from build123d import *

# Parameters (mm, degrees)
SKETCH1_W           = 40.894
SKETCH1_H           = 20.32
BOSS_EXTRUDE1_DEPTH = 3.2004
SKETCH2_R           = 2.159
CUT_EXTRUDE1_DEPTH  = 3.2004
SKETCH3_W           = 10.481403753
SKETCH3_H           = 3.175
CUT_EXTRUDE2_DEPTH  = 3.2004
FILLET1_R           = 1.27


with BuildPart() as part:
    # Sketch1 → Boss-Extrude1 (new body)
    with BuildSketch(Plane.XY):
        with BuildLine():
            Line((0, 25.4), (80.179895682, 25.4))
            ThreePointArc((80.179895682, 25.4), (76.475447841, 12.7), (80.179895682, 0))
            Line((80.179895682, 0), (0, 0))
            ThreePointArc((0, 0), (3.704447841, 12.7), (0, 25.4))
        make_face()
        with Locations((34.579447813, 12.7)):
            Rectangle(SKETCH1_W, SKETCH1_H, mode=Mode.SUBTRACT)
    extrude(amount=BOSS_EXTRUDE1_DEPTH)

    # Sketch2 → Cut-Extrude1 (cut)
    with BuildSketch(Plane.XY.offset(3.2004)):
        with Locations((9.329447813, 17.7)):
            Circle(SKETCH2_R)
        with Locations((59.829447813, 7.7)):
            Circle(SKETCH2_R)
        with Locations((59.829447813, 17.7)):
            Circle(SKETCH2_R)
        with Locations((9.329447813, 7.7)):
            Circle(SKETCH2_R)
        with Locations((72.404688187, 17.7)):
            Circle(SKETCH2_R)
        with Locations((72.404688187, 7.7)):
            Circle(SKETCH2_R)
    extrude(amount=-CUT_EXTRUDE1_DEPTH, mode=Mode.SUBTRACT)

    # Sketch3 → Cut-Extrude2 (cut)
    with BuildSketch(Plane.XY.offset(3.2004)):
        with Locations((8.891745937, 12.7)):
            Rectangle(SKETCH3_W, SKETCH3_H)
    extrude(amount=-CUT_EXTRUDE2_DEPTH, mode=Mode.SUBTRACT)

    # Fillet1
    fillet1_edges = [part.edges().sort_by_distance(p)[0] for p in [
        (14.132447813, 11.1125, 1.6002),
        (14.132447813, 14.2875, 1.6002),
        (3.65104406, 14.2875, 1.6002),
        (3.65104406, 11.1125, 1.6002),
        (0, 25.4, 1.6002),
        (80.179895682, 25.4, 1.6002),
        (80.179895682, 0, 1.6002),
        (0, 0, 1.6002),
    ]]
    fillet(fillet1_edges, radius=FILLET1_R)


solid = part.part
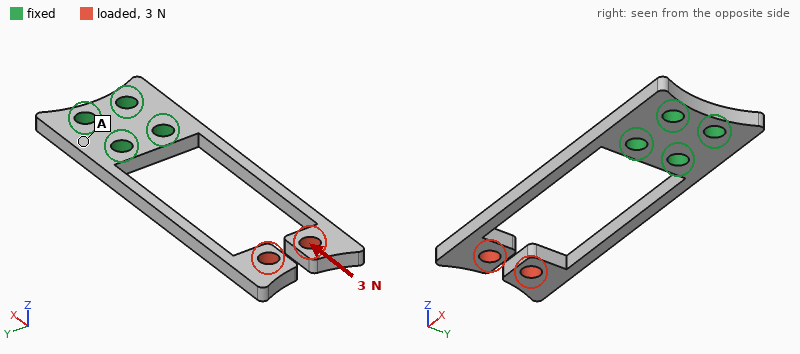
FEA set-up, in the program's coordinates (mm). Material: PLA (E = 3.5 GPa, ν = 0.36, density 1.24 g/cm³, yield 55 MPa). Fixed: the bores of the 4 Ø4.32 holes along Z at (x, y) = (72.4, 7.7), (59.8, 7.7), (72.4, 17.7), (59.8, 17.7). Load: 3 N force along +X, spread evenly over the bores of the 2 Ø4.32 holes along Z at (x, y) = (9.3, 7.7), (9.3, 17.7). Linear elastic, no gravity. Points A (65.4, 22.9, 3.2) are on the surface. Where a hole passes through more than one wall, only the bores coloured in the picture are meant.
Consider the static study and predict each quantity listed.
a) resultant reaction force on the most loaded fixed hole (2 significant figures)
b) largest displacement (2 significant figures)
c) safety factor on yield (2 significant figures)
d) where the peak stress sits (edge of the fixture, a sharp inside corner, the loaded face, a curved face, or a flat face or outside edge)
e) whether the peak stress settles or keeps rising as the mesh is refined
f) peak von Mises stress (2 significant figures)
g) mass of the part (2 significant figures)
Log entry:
1.6 N
0.92 mm
18
a flat face or outside edge
settles
3.0 MPa
3.8 g
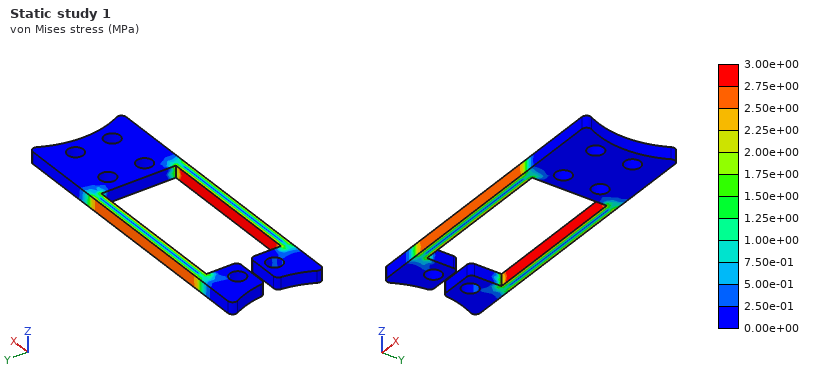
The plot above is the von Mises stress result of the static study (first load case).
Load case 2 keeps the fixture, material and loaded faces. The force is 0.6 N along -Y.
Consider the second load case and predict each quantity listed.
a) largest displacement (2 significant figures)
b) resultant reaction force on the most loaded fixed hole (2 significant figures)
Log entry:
0.87 mm
1.2 N
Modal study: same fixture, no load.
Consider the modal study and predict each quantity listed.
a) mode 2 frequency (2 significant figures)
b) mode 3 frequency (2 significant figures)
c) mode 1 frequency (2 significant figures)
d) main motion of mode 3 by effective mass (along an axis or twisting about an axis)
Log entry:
140 Hz
160 Hz
140 Hz
along Z
